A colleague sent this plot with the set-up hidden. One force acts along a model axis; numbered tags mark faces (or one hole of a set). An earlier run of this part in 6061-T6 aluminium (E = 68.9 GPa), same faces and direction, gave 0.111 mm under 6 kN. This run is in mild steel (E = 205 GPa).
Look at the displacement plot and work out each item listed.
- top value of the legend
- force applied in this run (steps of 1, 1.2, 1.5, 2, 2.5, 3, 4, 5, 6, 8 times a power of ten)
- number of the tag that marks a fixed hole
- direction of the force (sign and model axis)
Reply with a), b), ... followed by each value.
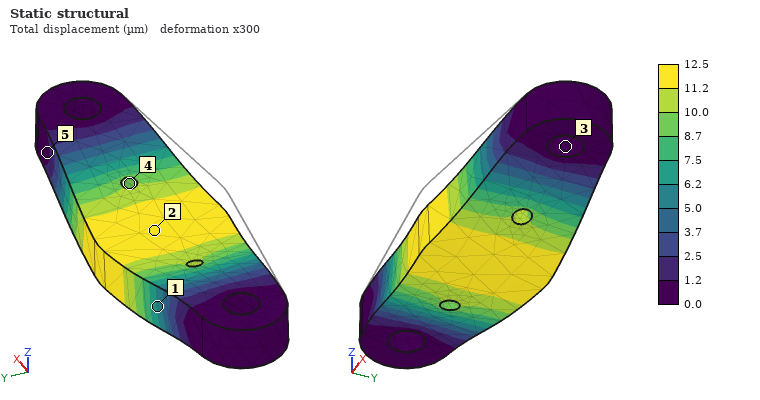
a) 12.5 µm
b) 2 kN
c) 3
d) -Z
